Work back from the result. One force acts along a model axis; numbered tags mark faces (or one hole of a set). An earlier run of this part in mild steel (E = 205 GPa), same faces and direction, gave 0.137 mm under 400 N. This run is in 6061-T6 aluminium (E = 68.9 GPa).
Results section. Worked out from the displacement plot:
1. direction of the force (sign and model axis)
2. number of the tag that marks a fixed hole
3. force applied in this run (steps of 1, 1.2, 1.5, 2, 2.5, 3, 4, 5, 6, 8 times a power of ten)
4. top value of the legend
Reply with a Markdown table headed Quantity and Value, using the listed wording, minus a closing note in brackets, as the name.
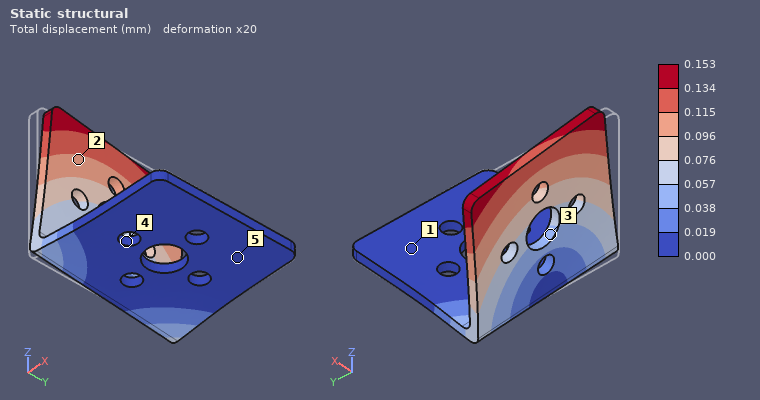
| Quantity | Value |
|---|---|
| direction of the force | +Y |
| number of the tag that marks a fixed hole | 4 |
| force applied in this run | 150 N |
| top value of the legend | 0.153 mm |
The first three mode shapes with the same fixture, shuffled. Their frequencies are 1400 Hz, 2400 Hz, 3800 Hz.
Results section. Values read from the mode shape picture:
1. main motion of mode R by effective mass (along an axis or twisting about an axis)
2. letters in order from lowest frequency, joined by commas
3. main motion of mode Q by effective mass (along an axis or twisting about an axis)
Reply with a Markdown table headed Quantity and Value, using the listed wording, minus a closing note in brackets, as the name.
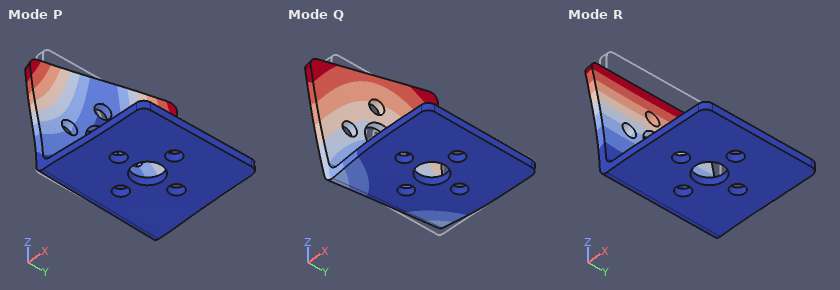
| Quantity | Value |
|---|---|
| main motion of mode R by effective mass | along X |
| letters in order from lowest frequency, joined by commas | R, Q, P |
| main motion of mode Q by effective mass | along Y |
